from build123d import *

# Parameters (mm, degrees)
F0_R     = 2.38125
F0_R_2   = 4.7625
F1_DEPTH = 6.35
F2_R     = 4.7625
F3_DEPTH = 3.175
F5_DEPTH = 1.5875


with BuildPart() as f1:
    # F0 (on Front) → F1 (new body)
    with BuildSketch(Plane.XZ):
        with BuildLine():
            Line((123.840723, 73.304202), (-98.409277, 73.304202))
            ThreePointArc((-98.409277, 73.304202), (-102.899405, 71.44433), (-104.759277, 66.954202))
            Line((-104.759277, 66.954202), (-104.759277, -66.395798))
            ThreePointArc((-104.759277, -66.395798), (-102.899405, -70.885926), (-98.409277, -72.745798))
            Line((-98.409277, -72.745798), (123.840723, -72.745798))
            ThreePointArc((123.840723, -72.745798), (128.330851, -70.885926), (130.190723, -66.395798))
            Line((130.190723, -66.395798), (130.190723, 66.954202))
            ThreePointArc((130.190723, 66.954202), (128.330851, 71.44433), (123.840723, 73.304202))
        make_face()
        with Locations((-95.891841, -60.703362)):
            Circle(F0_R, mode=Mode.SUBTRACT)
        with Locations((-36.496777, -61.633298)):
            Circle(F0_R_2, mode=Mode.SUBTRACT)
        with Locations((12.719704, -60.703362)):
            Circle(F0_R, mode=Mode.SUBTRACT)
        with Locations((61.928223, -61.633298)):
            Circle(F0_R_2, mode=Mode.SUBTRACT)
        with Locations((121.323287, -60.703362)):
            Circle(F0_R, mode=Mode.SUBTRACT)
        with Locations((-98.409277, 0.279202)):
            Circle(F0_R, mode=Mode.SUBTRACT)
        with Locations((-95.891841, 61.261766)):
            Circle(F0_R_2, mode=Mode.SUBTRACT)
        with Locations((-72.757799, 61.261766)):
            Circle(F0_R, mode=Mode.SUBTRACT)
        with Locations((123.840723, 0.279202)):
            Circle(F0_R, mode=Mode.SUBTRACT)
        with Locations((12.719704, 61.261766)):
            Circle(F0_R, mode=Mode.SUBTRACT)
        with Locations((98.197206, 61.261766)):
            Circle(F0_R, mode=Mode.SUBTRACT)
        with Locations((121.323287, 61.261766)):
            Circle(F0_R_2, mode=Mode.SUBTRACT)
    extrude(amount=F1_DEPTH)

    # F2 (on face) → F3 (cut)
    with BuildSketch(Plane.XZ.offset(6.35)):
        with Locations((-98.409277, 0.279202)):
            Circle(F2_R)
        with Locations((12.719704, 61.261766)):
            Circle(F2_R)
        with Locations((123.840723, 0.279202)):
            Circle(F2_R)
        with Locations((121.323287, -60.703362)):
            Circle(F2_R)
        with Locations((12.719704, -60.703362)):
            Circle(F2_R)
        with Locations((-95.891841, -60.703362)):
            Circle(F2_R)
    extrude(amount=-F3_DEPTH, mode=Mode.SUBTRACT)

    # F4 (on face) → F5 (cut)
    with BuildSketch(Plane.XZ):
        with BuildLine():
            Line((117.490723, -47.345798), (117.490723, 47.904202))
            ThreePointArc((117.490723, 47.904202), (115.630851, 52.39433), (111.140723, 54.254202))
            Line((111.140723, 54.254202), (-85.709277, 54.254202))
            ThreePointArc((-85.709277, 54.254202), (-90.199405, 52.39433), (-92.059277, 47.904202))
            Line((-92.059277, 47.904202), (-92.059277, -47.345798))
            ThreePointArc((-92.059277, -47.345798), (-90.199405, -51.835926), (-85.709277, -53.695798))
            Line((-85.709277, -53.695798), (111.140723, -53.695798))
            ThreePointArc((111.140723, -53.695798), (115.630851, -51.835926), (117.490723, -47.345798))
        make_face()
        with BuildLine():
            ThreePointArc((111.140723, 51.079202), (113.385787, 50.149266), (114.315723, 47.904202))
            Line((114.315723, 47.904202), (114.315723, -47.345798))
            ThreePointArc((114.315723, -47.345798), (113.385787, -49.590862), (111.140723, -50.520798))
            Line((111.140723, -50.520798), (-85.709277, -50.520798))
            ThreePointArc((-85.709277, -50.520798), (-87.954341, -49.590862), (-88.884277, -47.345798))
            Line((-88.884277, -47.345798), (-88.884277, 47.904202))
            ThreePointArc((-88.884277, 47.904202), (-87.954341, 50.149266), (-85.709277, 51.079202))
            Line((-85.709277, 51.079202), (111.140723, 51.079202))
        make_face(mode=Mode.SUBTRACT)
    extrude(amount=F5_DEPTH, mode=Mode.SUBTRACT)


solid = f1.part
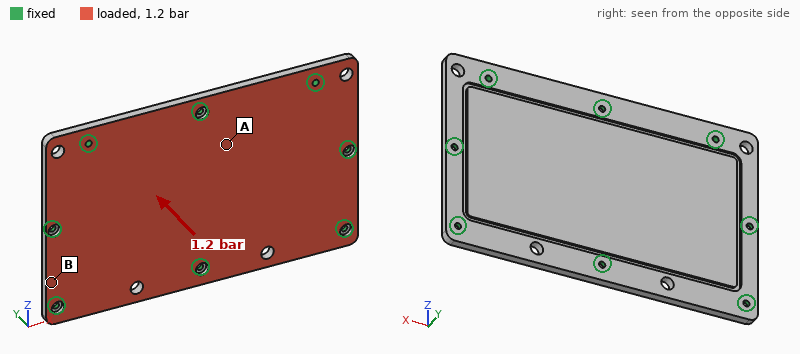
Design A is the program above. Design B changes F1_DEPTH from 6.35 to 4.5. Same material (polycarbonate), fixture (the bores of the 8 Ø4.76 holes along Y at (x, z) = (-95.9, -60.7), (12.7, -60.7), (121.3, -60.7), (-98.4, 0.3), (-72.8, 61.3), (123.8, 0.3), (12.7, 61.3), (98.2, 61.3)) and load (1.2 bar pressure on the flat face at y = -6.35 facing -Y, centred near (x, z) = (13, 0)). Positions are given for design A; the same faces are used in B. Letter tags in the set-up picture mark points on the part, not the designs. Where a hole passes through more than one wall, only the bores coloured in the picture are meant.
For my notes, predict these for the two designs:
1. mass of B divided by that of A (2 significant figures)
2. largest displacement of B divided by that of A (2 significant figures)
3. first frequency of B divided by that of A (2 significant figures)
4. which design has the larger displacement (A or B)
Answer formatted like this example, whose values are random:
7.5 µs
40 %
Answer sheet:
0.71
2.5
0.76
B
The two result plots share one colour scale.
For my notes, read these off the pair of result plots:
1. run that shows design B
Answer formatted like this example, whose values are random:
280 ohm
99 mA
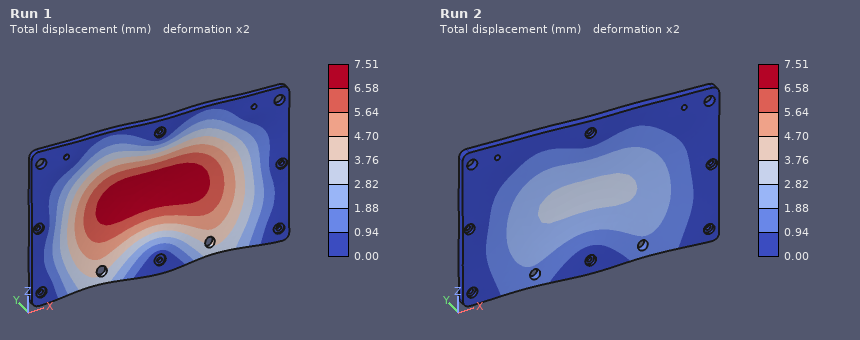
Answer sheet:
Run 1
